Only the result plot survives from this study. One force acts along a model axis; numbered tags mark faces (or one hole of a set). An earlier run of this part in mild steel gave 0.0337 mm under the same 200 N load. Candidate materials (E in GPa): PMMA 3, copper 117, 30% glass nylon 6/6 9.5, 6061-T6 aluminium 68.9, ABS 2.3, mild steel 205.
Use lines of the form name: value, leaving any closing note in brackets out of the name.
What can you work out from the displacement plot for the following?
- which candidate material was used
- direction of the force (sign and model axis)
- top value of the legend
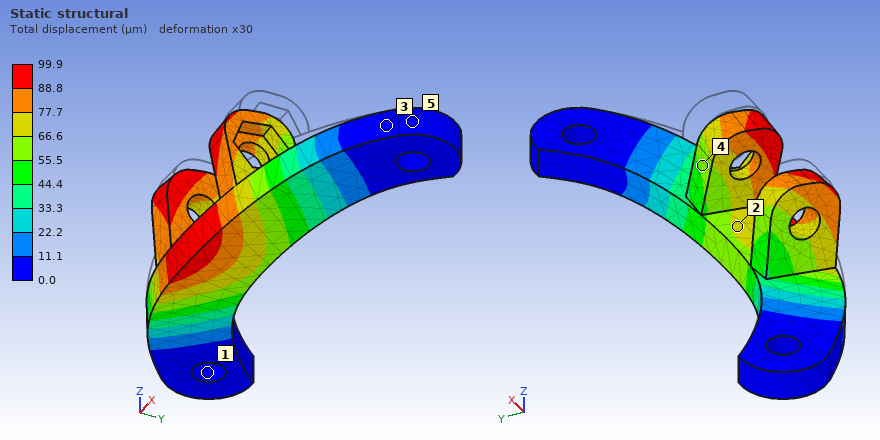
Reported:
which candidate material was used: 6061-T6 aluminium
direction of the force: -Z
top value of the legend: 99.9 µm
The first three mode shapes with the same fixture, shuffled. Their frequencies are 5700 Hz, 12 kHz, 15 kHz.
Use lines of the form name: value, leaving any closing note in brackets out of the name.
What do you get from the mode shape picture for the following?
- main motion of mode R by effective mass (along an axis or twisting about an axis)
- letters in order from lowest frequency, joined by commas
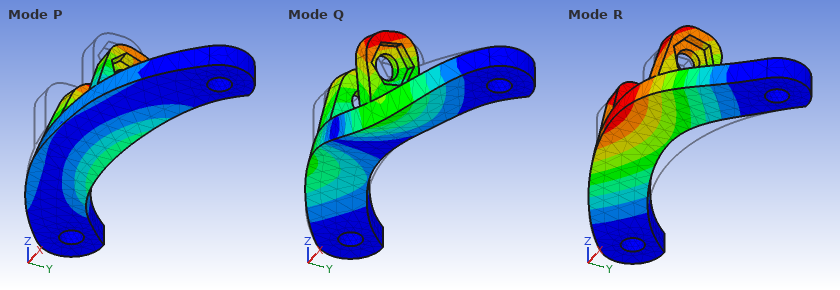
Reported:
main motion of mode R by effective mass: along Z
letters in order from lowest frequency, joined by commas: R, P, Q
